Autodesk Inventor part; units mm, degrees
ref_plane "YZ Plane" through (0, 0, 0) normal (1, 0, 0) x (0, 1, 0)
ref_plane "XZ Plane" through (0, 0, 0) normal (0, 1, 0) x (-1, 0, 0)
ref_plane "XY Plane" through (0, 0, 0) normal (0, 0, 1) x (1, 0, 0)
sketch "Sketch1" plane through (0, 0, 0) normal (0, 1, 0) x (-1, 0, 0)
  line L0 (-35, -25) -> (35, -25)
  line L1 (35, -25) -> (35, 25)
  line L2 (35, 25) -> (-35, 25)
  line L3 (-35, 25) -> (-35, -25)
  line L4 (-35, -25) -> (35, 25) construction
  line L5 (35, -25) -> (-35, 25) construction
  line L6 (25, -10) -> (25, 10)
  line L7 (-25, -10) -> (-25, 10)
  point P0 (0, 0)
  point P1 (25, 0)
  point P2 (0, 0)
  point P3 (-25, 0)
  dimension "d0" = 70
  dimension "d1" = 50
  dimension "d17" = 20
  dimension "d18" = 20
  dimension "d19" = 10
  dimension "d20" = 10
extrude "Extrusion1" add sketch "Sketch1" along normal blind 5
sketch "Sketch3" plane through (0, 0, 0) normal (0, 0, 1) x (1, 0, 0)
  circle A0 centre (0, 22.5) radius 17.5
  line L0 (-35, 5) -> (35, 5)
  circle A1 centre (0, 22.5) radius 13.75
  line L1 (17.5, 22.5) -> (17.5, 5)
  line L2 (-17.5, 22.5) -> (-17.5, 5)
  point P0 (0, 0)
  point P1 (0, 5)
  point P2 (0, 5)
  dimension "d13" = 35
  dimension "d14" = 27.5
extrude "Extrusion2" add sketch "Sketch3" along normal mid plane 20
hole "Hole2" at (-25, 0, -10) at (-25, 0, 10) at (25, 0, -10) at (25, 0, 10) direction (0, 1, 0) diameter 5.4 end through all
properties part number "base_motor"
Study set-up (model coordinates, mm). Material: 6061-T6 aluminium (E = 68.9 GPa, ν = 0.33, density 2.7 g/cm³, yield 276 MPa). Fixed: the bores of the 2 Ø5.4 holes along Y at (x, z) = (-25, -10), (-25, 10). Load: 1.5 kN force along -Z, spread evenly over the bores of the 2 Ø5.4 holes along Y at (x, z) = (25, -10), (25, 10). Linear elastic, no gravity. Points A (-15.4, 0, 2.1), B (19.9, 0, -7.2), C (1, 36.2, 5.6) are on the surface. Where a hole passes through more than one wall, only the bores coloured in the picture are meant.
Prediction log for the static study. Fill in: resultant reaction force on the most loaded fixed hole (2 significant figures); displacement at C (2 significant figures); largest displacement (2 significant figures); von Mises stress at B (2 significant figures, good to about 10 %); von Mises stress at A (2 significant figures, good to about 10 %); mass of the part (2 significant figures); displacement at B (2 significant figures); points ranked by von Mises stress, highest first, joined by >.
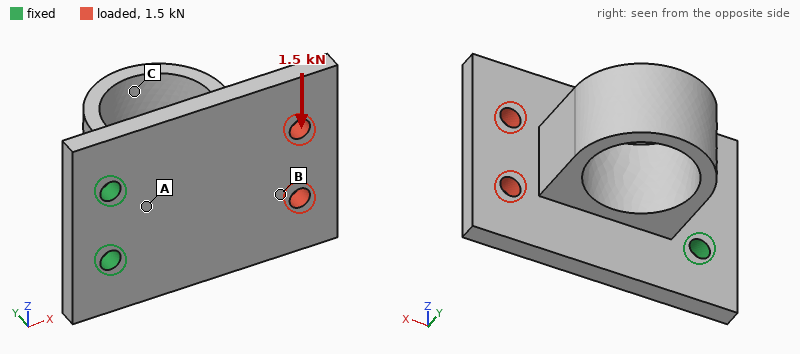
3.2 kN
11 µm
66 µm
16 MPa
30 MPa
73 g
44 µm
A > B > C
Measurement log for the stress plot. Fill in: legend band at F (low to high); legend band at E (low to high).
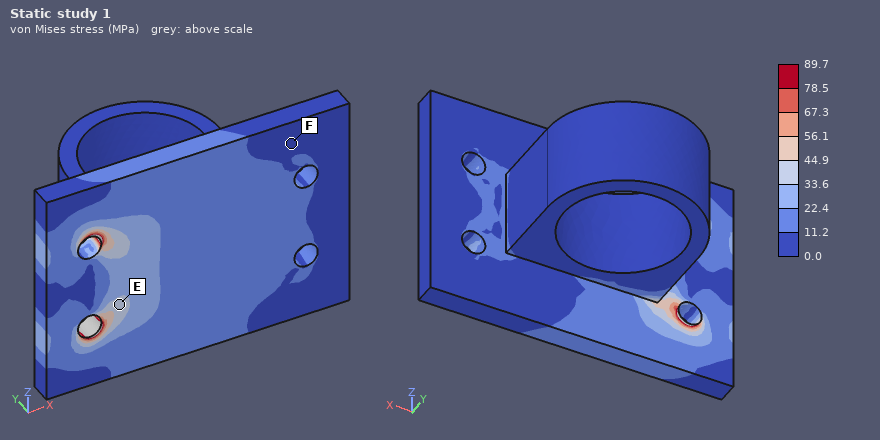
0.0 to 11.2 MPa
33.6 to 44.9 MPa
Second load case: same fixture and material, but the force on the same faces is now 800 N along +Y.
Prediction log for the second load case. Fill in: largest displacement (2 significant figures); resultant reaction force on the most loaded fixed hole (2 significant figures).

0.74 mm
420 N
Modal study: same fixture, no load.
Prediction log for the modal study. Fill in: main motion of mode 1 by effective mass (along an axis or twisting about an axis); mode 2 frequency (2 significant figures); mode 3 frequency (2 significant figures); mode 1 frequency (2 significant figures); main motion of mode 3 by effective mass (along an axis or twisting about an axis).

along Y
3400 Hz
5500 Hz
1100 Hz
along Z
